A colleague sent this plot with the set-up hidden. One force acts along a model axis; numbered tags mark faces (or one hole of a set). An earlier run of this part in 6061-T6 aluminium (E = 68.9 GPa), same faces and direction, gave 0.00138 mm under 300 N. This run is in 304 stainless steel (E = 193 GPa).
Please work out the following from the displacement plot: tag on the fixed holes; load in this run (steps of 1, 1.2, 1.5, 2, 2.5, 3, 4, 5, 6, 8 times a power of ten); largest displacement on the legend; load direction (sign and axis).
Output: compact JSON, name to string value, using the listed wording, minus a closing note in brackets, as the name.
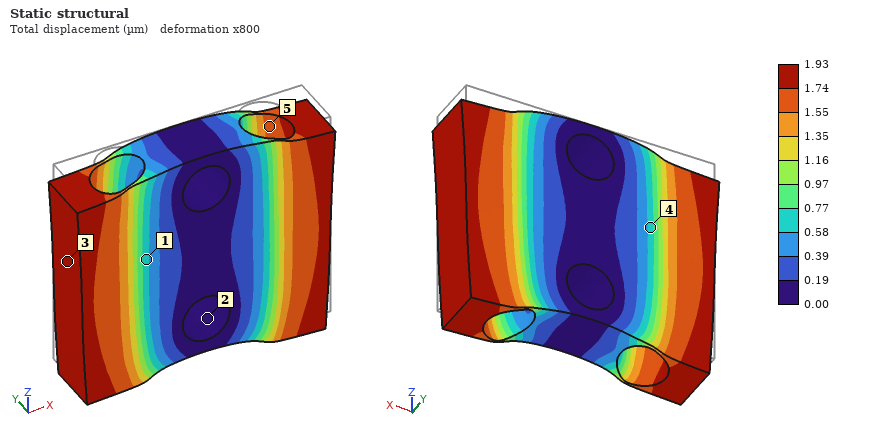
{"tag on the fixed holes": "2", "load in this run": "1.2 kN", "largest displacement on the legend": "1.93 µm", "load direction": "-Z"}
